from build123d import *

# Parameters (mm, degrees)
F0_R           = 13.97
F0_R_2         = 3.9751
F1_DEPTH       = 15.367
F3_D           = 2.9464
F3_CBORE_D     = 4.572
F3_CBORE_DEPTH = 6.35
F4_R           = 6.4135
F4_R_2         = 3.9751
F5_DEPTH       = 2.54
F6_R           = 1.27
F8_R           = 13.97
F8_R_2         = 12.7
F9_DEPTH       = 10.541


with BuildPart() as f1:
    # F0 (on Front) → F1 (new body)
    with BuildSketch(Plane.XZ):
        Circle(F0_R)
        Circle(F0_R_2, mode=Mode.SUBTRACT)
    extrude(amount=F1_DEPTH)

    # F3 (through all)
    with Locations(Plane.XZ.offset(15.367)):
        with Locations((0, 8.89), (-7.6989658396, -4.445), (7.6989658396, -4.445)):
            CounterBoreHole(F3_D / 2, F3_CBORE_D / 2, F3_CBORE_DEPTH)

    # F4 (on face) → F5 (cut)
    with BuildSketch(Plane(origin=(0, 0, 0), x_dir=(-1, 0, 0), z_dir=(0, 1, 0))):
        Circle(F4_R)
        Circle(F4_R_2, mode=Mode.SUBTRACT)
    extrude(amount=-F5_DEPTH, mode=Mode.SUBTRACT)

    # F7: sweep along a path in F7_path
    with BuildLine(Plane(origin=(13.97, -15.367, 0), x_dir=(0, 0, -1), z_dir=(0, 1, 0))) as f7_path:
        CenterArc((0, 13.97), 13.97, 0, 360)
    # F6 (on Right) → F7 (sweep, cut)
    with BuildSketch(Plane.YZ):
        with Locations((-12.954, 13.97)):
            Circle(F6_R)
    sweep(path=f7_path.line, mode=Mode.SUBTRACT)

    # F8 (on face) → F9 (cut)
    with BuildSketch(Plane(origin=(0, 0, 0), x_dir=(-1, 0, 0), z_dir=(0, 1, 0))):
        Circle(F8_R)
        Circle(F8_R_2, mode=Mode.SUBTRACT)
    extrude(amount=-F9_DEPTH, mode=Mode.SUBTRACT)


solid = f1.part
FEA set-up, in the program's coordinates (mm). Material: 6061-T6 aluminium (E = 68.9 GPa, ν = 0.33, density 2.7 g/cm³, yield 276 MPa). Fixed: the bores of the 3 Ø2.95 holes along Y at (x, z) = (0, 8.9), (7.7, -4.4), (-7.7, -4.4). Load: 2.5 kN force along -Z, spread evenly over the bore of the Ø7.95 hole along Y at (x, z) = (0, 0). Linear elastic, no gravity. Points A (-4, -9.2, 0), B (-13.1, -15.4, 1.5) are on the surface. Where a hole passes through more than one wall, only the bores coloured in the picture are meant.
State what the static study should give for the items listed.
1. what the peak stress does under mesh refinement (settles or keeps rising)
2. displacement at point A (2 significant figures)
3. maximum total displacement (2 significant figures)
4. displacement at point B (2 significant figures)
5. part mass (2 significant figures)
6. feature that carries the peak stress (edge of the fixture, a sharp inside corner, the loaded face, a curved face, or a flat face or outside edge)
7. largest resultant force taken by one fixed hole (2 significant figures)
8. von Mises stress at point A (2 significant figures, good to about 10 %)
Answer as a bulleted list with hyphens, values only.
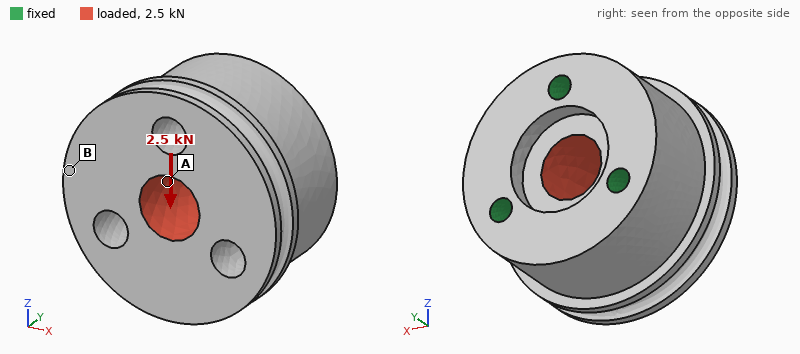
- keeps rising
- 1.7 µm
- 3.5 µm
- 1.6 µm
- 18 g
- edge of the fixture
- 900 N
- 19 MPa
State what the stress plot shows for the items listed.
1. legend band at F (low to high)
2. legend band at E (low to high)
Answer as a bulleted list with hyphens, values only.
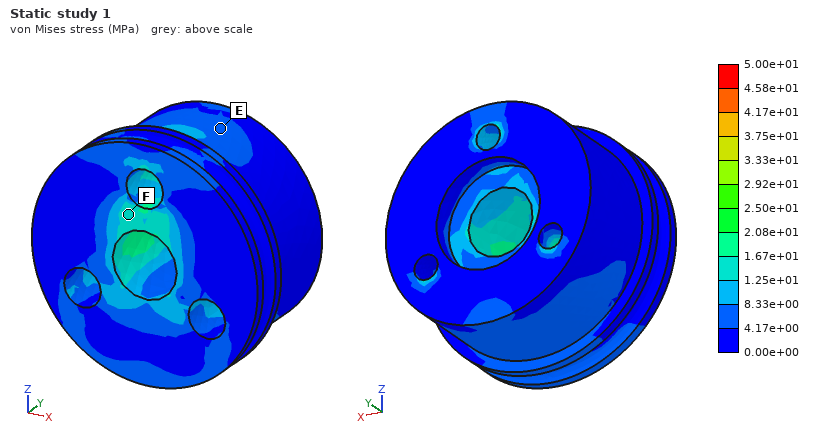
- 1.25e+01 to 1.67e+01 MPa
- 4.17e+00 to 8.33e+00 MPa
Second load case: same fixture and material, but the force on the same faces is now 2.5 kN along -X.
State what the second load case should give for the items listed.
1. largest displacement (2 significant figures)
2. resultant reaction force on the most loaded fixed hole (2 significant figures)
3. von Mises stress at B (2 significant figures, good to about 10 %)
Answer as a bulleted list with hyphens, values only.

- 3.2 µm
- 890 N
- 4.9 MPa
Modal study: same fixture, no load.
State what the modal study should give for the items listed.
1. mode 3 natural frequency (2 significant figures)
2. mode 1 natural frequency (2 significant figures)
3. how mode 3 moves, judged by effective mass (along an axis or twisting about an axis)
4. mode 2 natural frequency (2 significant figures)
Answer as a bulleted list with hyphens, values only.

- 58 kHz
- 41 kHz
- along Y
- 41 kHz
